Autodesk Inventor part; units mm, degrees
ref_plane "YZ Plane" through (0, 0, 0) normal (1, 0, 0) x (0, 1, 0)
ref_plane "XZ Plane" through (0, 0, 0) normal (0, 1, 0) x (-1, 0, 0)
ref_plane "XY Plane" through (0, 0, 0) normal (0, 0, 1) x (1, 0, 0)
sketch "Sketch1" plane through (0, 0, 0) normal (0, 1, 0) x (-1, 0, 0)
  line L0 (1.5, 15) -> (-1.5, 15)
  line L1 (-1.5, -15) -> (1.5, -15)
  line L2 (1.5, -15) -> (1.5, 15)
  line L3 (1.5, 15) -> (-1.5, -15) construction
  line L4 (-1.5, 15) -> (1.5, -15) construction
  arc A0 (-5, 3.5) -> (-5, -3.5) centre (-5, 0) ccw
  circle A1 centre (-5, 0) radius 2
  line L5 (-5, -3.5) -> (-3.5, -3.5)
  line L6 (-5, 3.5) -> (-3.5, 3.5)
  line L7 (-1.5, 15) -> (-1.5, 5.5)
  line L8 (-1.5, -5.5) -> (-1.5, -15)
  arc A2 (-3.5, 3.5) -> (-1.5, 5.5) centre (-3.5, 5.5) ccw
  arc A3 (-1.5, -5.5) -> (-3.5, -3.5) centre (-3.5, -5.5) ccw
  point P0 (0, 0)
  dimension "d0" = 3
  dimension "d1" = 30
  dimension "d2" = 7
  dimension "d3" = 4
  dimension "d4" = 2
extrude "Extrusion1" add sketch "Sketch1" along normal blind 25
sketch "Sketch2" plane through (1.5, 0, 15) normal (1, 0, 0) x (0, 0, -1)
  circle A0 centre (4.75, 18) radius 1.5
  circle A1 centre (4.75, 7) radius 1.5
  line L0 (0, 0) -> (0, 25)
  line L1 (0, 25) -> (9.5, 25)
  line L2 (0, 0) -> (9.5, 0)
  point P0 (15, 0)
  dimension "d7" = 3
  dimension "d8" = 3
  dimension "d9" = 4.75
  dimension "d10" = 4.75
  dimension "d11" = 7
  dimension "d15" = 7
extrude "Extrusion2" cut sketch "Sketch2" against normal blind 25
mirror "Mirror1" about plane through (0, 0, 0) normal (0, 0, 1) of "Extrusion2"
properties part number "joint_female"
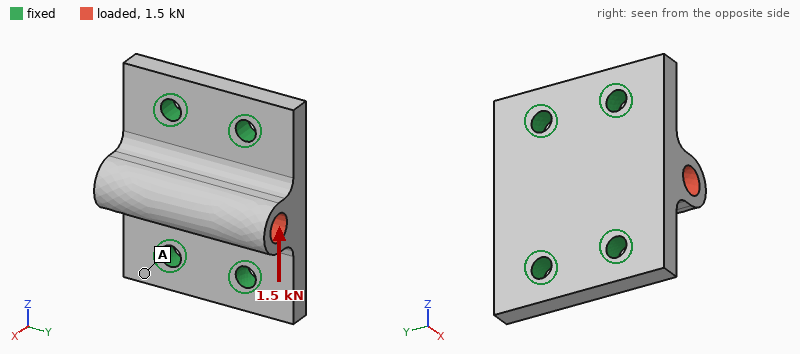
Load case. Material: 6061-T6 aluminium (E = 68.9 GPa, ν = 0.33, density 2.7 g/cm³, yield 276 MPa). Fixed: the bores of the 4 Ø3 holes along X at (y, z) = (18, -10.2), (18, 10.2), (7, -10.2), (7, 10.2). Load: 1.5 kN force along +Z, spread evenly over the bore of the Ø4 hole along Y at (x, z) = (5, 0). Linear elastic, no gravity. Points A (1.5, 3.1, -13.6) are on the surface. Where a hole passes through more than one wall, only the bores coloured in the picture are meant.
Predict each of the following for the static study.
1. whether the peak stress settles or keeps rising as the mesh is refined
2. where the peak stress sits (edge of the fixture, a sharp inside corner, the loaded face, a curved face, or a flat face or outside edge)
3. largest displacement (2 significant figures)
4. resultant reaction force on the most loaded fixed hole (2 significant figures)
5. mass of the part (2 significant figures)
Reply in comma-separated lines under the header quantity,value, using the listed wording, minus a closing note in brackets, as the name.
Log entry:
quantity,value
whether the peak stress settles or keeps rising as the mesh is refined,keeps rising
where the peak stress sits,edge of the fixture
largest displacement,13 µm
resultant reaction force on the most loaded fixed hole,450 N
mass of the part,8.1 g
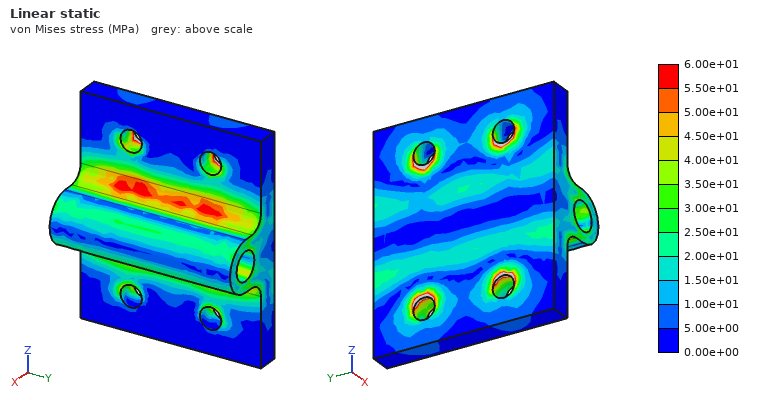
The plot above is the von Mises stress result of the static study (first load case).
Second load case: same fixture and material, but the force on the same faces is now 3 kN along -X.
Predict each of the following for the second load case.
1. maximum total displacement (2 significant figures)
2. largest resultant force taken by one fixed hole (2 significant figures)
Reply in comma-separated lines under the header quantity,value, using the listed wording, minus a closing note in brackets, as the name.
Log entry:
quantity,value
maximum total displacement,24 µm
largest resultant force taken by one fixed hole,810 N
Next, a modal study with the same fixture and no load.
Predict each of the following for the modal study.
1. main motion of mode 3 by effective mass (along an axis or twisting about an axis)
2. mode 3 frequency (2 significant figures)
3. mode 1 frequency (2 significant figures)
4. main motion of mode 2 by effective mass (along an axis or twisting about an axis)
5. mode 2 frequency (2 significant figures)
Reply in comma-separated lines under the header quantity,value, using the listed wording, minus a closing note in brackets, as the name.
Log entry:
quantity,value
main motion of mode 3 by effective mass,along Z
mode 3 frequency,42 kHz
mode 1 frequency,24 kHz
main motion of mode 2 by effective mass,along X
mode 2 frequency,29 kHz
